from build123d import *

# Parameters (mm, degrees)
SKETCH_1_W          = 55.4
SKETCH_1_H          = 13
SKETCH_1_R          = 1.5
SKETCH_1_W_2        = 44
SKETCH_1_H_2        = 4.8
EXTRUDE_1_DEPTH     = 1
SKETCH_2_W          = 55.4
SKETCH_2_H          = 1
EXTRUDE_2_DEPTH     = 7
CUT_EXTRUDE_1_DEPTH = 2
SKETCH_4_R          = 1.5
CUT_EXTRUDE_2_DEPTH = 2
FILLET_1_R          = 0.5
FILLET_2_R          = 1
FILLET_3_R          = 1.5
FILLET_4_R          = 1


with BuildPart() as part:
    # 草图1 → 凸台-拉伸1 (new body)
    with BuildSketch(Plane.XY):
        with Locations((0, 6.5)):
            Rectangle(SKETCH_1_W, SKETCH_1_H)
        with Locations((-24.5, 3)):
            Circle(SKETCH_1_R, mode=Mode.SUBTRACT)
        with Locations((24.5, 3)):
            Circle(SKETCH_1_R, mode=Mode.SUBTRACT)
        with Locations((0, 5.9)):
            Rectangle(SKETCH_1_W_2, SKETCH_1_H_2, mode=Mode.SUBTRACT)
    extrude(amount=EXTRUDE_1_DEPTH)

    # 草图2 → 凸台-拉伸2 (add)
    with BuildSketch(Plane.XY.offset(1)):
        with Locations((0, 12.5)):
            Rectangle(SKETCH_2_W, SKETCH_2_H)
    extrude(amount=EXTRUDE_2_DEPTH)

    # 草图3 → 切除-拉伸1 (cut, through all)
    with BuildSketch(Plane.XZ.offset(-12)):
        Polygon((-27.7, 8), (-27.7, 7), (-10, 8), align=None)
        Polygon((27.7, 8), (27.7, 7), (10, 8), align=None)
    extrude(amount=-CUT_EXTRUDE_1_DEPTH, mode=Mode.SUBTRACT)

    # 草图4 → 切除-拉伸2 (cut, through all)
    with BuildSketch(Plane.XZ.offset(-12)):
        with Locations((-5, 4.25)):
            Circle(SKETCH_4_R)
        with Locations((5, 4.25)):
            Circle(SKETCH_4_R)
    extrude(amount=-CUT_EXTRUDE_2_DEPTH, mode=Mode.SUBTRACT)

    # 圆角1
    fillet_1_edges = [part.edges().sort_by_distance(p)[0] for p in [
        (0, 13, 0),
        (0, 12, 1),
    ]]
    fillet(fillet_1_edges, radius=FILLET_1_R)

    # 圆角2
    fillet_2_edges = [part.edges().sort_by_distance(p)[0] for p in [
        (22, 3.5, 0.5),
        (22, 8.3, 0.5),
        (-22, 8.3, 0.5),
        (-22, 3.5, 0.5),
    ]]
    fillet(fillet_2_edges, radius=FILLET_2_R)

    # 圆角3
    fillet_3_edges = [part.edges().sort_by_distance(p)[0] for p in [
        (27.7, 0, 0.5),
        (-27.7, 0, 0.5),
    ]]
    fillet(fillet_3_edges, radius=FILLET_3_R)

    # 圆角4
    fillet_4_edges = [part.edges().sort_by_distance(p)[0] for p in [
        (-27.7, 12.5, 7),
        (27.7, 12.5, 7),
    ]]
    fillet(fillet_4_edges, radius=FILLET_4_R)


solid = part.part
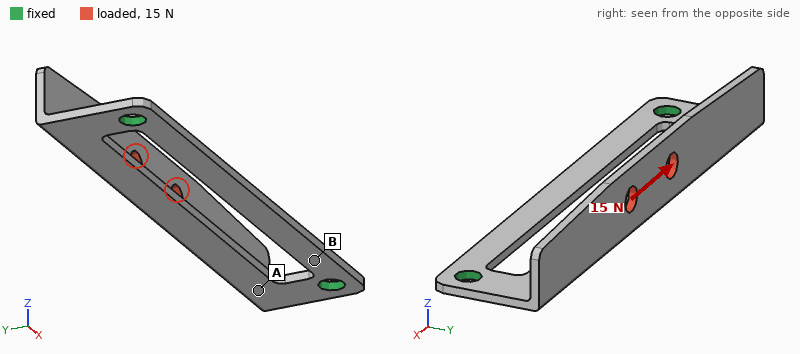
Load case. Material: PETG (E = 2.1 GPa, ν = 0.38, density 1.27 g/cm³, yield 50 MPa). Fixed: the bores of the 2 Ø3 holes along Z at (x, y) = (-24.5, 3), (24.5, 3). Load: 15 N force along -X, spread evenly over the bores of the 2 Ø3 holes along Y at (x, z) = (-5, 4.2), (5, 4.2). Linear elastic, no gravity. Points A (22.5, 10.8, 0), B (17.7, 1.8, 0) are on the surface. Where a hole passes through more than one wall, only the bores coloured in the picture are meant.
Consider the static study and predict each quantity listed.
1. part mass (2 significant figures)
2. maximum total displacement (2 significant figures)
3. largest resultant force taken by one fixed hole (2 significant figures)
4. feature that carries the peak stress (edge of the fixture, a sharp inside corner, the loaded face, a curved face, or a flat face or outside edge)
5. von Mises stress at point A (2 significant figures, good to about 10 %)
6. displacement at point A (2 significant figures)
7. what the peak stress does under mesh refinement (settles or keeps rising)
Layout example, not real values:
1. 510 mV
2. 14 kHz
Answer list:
1. 1.1 g
2. 0.20 mm
3. 7.7 N
4. edge of the fixture
5. 1.6 MPa
6. 0.090 mm
7. keeps rising
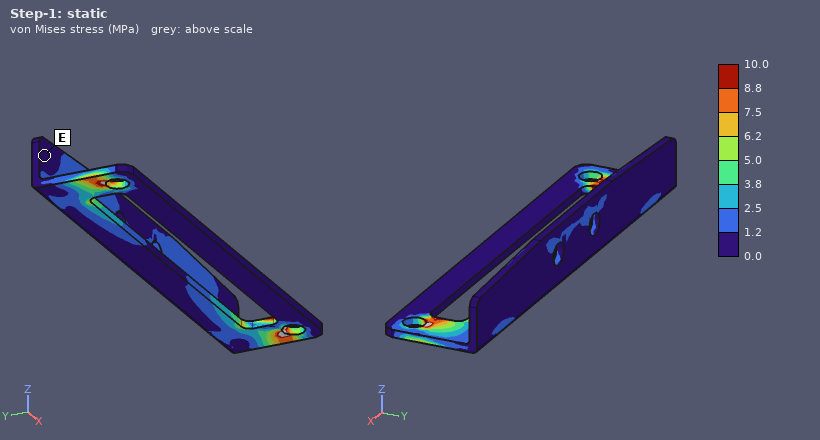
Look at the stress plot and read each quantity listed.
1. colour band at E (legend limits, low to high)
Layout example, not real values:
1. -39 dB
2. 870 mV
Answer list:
1. 0.0 to 1.2 MPa
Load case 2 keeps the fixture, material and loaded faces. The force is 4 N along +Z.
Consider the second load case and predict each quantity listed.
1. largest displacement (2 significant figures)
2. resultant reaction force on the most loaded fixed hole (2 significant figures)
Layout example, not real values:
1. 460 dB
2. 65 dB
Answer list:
1. 0.68 mm
2. 2.0 N
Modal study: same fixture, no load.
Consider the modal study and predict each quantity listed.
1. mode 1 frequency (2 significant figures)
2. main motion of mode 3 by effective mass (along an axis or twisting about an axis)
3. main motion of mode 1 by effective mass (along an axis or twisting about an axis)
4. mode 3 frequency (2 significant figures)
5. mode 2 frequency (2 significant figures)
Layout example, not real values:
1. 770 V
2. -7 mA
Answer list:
1. 540 Hz
2. twisting about Y
3. along Z
4. 1100 Hz
5. 620 Hz
